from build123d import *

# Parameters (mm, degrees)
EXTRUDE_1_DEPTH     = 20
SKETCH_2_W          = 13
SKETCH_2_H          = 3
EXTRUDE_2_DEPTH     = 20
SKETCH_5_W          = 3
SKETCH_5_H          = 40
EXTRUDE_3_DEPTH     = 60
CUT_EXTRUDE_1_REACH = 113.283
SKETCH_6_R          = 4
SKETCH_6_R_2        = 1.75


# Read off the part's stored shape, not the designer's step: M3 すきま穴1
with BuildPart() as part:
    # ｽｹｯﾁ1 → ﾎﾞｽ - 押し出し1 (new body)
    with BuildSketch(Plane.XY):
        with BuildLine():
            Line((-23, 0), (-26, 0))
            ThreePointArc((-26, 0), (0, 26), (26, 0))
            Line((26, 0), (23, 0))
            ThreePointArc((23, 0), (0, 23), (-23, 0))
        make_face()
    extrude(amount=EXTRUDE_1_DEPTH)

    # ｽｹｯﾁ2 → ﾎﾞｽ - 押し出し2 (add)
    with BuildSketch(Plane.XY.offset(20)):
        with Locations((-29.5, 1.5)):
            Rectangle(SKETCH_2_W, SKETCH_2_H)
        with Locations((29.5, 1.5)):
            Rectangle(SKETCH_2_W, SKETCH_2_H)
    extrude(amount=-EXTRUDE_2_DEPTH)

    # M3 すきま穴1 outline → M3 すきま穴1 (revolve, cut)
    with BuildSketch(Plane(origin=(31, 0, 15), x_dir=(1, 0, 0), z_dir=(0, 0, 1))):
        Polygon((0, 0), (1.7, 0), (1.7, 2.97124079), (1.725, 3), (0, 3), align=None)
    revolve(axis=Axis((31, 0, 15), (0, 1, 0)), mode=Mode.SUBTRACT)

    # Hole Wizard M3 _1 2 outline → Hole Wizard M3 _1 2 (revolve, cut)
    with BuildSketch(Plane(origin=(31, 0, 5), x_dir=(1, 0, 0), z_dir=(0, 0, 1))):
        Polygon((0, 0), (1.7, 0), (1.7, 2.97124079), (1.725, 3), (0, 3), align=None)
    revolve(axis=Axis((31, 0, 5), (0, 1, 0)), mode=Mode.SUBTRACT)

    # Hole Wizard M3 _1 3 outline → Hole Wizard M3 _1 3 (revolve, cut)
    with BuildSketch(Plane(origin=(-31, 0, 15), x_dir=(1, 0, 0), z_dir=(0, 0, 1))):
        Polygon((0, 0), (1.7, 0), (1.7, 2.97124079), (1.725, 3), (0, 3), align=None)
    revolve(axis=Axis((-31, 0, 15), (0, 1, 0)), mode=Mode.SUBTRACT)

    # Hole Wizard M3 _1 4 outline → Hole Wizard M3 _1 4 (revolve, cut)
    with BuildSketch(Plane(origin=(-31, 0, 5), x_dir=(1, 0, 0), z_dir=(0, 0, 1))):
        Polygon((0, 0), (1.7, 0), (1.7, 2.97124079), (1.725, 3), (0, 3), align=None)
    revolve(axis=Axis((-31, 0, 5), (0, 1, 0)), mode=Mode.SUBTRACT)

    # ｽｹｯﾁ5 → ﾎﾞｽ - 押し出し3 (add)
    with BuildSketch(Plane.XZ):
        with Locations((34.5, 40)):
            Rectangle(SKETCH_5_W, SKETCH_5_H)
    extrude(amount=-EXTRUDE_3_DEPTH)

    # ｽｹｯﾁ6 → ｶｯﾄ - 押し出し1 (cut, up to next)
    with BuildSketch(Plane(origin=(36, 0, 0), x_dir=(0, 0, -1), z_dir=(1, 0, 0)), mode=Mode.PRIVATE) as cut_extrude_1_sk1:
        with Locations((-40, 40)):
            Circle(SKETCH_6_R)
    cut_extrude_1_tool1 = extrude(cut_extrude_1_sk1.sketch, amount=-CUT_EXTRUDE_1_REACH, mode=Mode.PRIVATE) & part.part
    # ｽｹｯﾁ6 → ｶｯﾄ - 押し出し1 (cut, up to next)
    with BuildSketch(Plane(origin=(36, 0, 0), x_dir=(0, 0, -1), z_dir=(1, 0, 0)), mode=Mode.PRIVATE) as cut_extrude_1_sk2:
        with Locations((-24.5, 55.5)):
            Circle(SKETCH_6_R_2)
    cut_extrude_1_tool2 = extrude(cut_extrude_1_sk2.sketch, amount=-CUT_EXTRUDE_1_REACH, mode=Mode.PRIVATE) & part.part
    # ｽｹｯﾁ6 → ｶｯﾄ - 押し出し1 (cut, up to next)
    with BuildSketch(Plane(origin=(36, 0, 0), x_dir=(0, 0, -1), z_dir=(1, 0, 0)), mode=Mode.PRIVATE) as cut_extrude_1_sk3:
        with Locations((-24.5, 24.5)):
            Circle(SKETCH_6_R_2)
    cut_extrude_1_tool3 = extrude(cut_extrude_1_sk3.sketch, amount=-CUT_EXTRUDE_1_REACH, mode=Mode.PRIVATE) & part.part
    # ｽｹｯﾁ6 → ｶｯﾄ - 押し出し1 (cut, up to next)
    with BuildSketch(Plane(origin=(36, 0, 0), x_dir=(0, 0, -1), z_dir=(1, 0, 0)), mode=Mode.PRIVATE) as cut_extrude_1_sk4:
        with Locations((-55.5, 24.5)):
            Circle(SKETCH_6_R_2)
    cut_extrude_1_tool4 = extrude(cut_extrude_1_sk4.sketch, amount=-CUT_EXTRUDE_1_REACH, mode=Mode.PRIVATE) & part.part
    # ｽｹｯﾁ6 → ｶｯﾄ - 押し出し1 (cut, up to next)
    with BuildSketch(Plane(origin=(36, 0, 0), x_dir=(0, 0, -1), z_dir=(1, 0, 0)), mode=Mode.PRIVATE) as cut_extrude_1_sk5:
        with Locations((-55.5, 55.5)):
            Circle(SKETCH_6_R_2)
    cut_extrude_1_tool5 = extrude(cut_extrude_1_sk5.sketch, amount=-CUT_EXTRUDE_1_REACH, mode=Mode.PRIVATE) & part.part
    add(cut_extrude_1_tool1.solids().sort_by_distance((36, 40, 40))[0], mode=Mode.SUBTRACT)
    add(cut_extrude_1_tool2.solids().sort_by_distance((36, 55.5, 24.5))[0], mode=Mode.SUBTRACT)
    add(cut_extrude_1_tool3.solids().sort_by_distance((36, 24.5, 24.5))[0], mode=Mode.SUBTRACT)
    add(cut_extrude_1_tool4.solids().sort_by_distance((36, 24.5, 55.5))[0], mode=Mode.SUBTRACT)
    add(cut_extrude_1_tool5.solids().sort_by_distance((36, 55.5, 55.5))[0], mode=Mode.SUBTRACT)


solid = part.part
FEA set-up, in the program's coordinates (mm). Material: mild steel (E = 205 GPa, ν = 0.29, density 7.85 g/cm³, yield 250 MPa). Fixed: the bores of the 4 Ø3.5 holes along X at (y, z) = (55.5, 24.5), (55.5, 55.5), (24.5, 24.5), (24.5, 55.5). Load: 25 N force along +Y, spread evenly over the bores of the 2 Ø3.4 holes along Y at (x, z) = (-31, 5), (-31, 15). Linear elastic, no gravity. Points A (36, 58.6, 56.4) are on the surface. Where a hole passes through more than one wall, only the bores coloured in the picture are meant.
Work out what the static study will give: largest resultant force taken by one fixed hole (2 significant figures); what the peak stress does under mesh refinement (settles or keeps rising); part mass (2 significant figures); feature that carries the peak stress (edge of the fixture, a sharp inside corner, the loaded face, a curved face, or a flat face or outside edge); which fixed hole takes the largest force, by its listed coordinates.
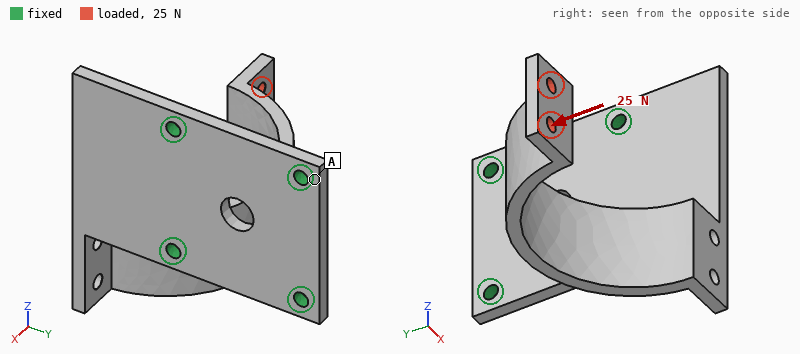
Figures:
36 N
keeps rising
99 g
a sharp inside corner
(24.5, 24.5)
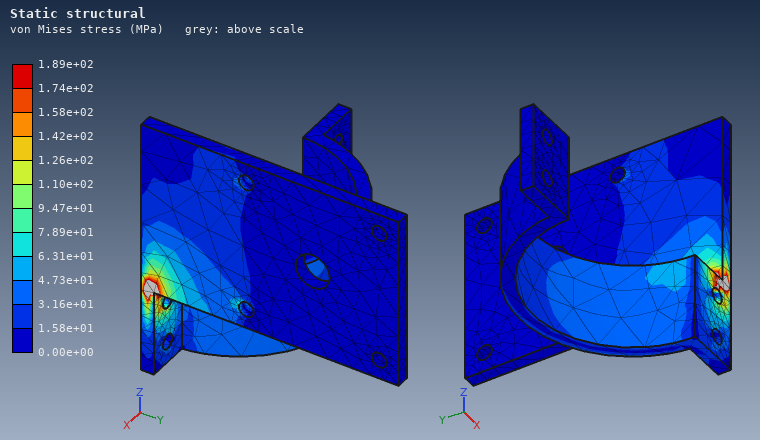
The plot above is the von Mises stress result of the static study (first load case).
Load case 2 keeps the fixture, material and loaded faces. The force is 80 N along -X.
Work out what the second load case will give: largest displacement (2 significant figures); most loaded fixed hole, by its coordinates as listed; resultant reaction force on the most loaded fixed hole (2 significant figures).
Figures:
0.70 mm
(24.5, 24.5)
120 N
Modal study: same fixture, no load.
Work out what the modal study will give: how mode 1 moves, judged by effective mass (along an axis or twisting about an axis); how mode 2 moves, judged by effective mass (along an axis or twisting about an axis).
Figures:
along Y
along Z
